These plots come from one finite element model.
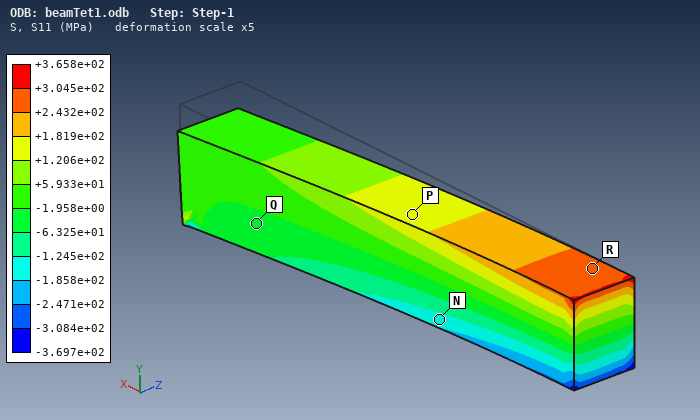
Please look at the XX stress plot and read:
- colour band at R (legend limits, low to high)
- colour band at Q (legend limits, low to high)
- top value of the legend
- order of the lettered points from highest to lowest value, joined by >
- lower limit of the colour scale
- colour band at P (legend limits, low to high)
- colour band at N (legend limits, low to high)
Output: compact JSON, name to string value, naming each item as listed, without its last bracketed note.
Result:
{"colour band at R": "+2.432e+02 to +3.045e+02 MPa", "colour band at Q": "-6.325e+01 to -1.958e+00 MPa", "top value of the legend": "+3.658e+02 MPa", "order of the lettered points from highest to lowest value, joined by >": "R > P > Q > N", "lower limit of the colour scale": "-3.697e+02 MPa", "colour band at P": "+1.206e+02 to +1.819e+02 MPa", "colour band at N": "-1.858e+02 to -1.245e+02 MPa"}
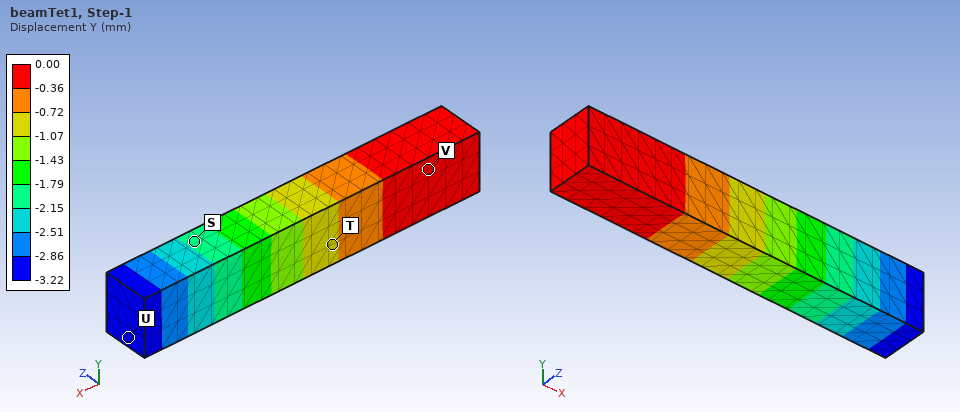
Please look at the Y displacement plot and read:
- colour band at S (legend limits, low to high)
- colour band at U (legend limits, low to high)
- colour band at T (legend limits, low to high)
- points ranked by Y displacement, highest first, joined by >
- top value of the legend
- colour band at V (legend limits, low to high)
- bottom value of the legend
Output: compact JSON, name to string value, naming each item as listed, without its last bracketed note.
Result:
{"colour band at S": "-2.15 to -1.79 mm", "colour band at U": "-3.22 to -2.86 mm", "colour band at T": "-1.07 to -0.72 mm", "points ranked by Y displacement, highest first, joined by >": "V > T > S > U", "top value of the legend": "0.00 mm", "colour band at V": "-0.36 to 0.00 mm", "bottom value of the legend": "-3.22 mm"}
